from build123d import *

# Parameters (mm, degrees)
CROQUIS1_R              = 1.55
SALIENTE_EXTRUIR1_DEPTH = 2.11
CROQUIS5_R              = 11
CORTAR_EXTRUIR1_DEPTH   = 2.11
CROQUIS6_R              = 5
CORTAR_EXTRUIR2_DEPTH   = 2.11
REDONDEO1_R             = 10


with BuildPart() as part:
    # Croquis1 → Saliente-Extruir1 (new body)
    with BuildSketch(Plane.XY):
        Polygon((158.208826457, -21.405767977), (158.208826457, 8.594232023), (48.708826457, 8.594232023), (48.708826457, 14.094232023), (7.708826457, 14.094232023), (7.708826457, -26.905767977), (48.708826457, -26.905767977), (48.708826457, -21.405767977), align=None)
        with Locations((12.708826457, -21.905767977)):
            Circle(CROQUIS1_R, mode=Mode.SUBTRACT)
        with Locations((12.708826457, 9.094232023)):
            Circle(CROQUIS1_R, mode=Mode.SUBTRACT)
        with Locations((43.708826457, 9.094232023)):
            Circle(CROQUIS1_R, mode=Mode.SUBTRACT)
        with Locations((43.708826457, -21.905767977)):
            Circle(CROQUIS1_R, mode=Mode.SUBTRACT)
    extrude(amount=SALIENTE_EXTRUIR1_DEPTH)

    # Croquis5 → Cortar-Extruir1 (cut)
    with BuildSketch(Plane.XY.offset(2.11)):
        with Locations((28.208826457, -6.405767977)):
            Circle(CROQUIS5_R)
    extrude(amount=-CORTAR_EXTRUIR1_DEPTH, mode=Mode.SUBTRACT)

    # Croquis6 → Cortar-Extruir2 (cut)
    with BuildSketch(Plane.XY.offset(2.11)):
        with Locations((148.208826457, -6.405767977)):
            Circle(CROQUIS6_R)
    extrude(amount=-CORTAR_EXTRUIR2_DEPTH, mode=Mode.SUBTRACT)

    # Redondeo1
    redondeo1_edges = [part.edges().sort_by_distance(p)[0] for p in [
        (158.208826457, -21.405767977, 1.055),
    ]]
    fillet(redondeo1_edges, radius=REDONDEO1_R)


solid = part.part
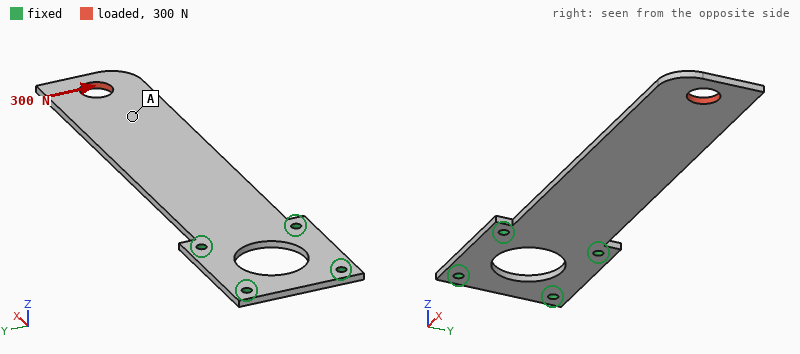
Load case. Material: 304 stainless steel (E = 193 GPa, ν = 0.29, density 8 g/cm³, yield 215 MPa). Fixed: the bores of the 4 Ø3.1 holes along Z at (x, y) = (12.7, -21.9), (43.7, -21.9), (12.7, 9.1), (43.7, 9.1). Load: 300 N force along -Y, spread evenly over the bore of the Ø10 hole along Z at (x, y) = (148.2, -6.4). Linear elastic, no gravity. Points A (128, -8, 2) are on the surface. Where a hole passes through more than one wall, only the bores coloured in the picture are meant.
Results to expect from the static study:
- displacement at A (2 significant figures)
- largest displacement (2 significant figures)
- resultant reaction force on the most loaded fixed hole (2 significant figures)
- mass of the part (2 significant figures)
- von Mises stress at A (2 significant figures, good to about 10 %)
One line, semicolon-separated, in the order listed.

0.096 mm; 0.16 mm; 1.0 kN; 75 g; 13 MPa
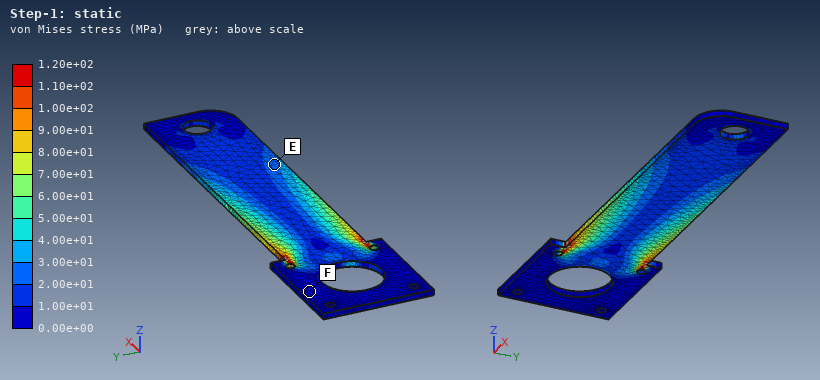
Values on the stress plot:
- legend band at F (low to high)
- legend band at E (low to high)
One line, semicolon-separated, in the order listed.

0.00e+00 to 1.00e+01 MPa; 2.00e+01 to 3.00e+01 MPa
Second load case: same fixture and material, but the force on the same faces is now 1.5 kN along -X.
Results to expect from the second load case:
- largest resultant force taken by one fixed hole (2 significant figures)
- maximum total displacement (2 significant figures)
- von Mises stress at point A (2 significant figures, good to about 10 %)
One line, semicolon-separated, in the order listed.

720 N; 18 µm; 24 MPa
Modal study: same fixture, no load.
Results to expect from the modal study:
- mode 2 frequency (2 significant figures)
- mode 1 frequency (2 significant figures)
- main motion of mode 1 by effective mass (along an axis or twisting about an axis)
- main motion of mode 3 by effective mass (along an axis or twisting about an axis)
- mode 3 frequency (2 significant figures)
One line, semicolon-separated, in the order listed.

800 Hz; 130 Hz; along Z; twisting about X; 1000 Hz
